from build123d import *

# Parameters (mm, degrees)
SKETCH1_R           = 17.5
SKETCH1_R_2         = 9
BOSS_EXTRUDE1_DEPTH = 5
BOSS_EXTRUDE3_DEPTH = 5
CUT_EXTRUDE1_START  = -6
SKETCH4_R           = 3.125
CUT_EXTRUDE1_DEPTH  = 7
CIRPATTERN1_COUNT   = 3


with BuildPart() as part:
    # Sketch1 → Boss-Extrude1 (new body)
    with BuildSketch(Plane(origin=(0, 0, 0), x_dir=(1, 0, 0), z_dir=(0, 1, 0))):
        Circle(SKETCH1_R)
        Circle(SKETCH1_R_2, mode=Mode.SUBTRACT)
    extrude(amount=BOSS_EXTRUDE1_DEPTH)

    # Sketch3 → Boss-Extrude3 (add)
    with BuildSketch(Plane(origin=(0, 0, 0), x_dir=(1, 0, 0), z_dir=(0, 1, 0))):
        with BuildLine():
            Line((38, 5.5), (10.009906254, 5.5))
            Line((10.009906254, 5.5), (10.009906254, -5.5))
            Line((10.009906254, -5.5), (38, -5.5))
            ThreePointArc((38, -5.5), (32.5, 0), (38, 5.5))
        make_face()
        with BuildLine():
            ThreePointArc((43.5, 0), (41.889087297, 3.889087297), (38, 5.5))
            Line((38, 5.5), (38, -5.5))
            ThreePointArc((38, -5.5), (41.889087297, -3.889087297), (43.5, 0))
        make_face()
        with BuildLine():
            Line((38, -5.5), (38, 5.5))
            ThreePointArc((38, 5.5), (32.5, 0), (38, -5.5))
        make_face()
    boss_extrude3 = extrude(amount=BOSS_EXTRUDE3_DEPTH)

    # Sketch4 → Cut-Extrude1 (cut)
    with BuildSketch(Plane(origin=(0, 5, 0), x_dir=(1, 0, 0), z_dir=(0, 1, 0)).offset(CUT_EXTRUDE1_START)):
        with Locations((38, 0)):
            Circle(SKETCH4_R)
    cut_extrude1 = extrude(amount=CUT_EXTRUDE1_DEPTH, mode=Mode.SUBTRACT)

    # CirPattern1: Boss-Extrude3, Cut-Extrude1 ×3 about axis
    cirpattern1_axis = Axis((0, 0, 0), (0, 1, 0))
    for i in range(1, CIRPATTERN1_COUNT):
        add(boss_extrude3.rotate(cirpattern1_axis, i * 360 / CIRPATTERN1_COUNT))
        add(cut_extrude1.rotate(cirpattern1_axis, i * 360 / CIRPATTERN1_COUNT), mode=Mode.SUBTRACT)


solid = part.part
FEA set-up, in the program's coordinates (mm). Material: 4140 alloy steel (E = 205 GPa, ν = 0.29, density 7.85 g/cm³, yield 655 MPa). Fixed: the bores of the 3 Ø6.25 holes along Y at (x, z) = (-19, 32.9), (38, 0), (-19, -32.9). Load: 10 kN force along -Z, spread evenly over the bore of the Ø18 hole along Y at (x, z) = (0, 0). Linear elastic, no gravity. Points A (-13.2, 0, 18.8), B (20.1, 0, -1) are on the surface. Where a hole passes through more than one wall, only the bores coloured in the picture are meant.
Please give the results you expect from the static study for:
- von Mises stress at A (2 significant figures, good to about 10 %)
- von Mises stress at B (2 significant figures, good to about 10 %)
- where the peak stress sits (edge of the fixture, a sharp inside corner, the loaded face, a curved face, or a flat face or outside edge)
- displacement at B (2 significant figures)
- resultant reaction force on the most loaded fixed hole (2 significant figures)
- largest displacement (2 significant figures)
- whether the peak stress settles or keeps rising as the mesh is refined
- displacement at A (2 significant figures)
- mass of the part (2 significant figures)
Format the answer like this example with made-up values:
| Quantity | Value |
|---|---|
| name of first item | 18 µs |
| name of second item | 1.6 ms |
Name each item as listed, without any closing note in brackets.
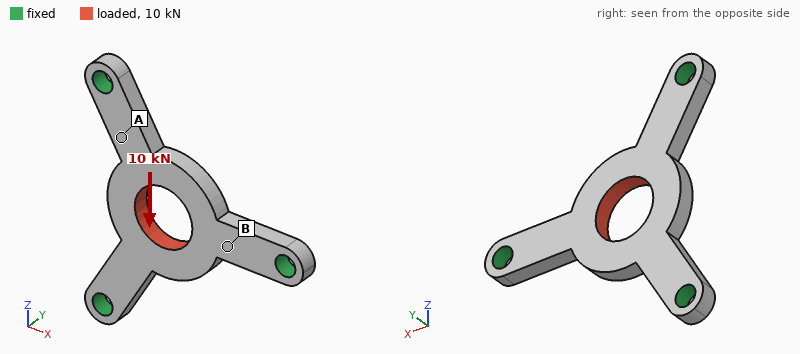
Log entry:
| Quantity | Value |
|---|---|
| von Mises stress at A | 86 MPa |
| von Mises stress at B | 43 MPa |
| where the peak stress sits | a sharp inside corner |
| displacement at B | 21 µm |
| resultant reaction force on the most loaded fixed hole | 4.9 kN |
| largest displacement | 38 µm |
| whether the peak stress settles or keeps rising as the mesh is refined | keeps rising |
| displacement at A | 9.1 µm |
| mass of the part | 57 g |
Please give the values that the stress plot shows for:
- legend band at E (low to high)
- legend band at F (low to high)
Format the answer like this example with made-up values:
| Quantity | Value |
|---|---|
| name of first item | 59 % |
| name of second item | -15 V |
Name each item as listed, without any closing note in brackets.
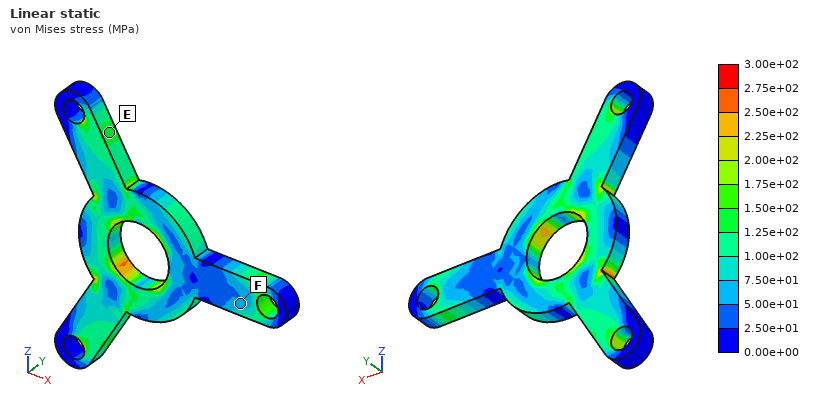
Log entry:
| Quantity | Value |
|---|---|
| legend band at E | 1.25e+02 to 1.50e+02 MPa |
| legend band at F | 5.00e+01 to 7.50e+01 MPa |
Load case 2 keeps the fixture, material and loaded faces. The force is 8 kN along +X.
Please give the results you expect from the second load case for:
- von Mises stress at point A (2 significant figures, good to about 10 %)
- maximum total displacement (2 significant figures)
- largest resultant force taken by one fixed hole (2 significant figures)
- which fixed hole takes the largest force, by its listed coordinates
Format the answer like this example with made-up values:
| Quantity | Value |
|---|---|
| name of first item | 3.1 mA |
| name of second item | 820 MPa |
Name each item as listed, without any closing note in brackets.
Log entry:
| Quantity | Value |
|---|---|
| von Mises stress at point A | 56 MPa |
| maximum total displacement | 32 µm |
| largest resultant force taken by one fixed hole | 4.6 kN |
| which fixed hole takes the largest force, by its listed coordinates | (38, 0) |
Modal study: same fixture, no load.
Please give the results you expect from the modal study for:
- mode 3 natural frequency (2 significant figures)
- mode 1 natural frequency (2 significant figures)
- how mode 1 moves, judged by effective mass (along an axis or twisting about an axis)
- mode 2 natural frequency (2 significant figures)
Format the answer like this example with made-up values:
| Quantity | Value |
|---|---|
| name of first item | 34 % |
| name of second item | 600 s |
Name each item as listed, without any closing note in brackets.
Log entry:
| Quantity | Value |
|---|---|
| mode 3 natural frequency | 9600 Hz |
| mode 1 natural frequency | 5300 Hz |
| how mode 1 moves, judged by effective mass | along Y |
| mode 2 natural frequency | 9600 Hz |
